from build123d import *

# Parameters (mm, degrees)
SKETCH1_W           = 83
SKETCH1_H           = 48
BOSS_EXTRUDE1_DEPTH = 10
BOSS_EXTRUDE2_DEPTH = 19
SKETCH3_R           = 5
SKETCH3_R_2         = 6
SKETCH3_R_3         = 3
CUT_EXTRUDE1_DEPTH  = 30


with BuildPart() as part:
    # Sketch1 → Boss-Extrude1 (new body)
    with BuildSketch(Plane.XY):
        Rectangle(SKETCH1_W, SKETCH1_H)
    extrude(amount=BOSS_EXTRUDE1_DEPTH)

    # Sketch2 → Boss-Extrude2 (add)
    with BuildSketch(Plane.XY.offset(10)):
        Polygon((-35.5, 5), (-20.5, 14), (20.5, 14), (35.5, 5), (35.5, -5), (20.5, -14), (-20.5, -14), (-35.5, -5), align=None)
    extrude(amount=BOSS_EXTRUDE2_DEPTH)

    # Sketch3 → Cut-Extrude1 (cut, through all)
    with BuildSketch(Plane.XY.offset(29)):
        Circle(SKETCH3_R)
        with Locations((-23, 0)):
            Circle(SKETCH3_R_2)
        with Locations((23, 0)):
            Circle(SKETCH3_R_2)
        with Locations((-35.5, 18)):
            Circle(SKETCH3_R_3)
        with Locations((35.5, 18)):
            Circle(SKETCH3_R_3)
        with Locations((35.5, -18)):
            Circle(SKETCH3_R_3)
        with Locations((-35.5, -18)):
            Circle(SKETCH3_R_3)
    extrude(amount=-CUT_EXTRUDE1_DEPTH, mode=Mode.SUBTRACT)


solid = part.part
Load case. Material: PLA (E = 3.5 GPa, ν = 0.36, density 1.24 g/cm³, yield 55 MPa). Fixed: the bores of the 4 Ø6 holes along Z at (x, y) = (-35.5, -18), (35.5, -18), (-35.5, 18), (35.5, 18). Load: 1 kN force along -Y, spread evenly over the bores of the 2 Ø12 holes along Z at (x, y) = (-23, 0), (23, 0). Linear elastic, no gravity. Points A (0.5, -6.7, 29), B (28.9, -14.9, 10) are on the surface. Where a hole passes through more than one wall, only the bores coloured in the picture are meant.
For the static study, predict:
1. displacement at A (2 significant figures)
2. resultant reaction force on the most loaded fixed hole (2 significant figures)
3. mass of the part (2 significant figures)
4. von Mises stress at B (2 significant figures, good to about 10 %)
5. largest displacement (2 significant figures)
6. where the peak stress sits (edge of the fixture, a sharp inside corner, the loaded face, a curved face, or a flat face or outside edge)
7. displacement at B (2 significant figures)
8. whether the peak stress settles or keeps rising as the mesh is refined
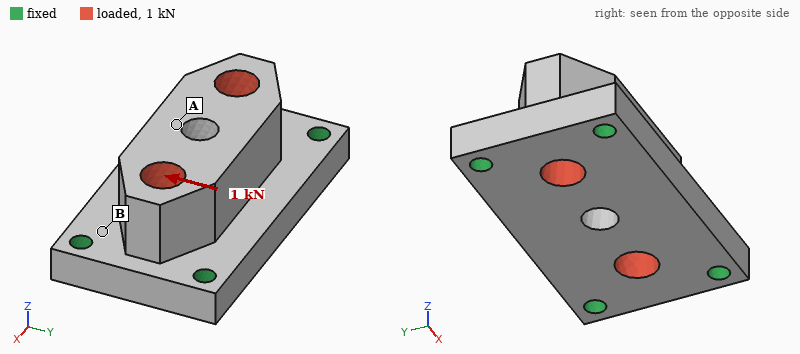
44 µm
320 N
78 g
2.9 MPa
49 µm
edge of the fixture
8.2 µm
keeps rising
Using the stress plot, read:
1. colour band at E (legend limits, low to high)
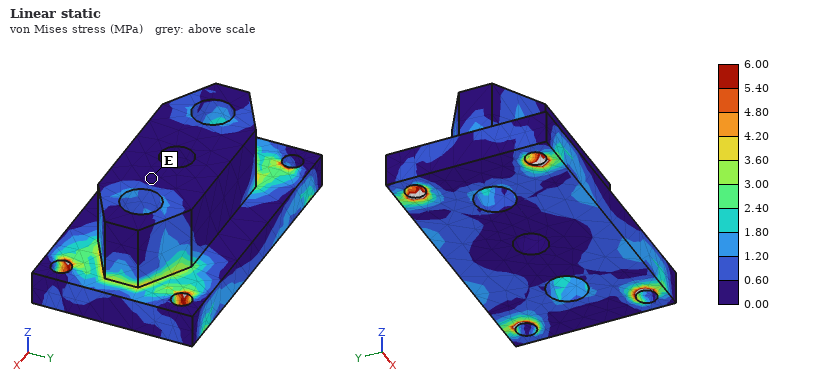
0.00 to 0.60 MPa
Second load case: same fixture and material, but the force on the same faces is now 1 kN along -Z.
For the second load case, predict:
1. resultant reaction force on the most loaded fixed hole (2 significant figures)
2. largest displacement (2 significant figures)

260 N
34 µm
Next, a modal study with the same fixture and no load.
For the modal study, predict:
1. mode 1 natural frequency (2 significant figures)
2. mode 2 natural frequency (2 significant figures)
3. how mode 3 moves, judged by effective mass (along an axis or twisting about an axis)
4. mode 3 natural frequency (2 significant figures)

3100 Hz
3200 Hz
along Y
4800 Hz
